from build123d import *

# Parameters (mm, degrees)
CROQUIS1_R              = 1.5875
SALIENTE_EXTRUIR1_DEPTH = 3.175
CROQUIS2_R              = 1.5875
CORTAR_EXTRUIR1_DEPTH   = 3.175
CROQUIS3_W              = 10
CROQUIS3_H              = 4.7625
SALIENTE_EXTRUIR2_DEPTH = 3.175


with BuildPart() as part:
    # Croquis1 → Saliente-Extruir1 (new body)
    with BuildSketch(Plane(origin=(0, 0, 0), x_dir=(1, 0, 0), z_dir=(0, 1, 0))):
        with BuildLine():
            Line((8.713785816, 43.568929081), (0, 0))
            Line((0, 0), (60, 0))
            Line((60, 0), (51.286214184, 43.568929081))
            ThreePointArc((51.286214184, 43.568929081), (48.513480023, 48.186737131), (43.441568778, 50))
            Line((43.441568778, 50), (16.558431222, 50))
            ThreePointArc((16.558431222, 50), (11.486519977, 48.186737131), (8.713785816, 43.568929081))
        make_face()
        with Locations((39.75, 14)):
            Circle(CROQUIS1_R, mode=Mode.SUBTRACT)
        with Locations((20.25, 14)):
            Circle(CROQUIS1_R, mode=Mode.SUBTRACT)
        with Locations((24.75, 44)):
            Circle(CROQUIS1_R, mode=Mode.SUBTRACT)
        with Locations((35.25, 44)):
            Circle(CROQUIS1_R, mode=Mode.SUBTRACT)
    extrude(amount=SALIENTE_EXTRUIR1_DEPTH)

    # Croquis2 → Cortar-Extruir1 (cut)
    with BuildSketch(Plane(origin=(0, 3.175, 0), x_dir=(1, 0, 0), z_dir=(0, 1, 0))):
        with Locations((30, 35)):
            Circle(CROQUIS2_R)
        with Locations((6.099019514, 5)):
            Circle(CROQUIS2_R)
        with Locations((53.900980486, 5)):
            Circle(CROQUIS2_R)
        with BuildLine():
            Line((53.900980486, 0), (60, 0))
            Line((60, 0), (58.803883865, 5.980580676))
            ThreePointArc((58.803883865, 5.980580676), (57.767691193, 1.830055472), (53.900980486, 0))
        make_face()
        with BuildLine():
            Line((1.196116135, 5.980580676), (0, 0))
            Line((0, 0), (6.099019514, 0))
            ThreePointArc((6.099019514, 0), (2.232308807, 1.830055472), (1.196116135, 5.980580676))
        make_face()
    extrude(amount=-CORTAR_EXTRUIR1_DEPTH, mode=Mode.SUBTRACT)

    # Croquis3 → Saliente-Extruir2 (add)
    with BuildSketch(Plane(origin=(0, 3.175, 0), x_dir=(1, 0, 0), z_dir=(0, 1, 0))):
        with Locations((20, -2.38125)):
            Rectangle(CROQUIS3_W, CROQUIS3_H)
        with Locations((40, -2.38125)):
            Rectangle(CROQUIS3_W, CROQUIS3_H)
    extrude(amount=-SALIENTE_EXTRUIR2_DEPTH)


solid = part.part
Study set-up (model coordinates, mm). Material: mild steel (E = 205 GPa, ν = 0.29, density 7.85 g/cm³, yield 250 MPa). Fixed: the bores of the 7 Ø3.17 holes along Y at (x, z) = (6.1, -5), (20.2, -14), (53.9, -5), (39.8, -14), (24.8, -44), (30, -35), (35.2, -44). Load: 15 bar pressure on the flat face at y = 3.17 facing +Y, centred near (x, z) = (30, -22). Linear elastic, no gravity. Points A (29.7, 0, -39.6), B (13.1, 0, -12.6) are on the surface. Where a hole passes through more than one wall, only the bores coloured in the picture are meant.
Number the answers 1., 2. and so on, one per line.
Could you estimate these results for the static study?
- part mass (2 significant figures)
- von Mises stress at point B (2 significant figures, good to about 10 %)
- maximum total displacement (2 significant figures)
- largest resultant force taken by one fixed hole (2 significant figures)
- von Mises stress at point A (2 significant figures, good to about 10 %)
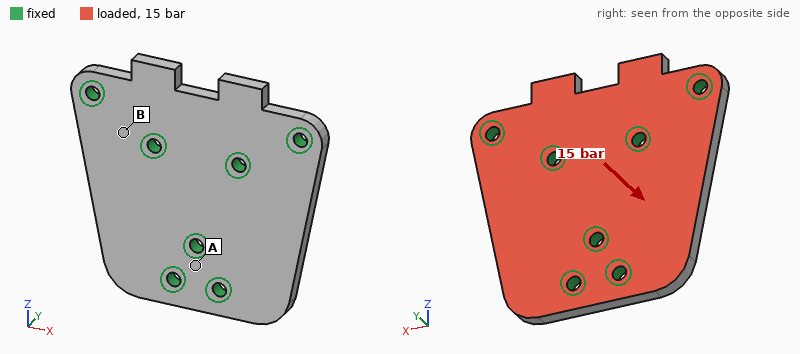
1. 62 g
2. 56 MPa
3. 28 µm
4. 770 N
5. 21 MPa
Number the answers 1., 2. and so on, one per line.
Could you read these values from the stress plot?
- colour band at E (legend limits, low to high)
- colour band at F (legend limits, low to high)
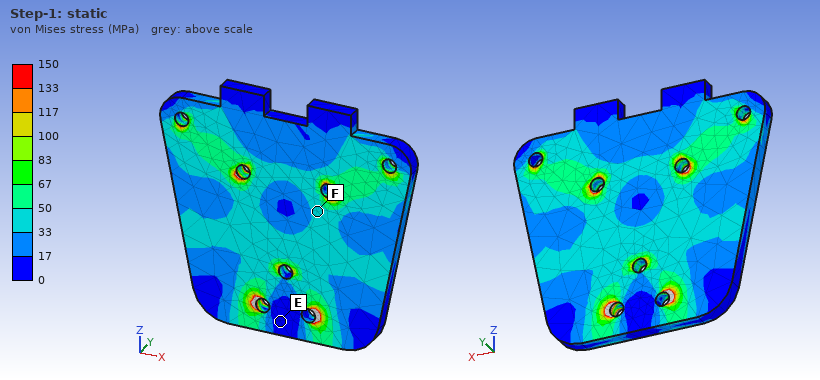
1. 0 to 17 MPa
2. 33 to 50 MPa
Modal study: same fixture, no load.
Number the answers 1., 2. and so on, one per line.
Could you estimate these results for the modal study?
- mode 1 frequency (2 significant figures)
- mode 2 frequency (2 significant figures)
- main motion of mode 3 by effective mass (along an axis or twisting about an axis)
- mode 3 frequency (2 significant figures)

1. 9700 Hz
2. 9700 Hz
3. along Y
4. 12 kHz
